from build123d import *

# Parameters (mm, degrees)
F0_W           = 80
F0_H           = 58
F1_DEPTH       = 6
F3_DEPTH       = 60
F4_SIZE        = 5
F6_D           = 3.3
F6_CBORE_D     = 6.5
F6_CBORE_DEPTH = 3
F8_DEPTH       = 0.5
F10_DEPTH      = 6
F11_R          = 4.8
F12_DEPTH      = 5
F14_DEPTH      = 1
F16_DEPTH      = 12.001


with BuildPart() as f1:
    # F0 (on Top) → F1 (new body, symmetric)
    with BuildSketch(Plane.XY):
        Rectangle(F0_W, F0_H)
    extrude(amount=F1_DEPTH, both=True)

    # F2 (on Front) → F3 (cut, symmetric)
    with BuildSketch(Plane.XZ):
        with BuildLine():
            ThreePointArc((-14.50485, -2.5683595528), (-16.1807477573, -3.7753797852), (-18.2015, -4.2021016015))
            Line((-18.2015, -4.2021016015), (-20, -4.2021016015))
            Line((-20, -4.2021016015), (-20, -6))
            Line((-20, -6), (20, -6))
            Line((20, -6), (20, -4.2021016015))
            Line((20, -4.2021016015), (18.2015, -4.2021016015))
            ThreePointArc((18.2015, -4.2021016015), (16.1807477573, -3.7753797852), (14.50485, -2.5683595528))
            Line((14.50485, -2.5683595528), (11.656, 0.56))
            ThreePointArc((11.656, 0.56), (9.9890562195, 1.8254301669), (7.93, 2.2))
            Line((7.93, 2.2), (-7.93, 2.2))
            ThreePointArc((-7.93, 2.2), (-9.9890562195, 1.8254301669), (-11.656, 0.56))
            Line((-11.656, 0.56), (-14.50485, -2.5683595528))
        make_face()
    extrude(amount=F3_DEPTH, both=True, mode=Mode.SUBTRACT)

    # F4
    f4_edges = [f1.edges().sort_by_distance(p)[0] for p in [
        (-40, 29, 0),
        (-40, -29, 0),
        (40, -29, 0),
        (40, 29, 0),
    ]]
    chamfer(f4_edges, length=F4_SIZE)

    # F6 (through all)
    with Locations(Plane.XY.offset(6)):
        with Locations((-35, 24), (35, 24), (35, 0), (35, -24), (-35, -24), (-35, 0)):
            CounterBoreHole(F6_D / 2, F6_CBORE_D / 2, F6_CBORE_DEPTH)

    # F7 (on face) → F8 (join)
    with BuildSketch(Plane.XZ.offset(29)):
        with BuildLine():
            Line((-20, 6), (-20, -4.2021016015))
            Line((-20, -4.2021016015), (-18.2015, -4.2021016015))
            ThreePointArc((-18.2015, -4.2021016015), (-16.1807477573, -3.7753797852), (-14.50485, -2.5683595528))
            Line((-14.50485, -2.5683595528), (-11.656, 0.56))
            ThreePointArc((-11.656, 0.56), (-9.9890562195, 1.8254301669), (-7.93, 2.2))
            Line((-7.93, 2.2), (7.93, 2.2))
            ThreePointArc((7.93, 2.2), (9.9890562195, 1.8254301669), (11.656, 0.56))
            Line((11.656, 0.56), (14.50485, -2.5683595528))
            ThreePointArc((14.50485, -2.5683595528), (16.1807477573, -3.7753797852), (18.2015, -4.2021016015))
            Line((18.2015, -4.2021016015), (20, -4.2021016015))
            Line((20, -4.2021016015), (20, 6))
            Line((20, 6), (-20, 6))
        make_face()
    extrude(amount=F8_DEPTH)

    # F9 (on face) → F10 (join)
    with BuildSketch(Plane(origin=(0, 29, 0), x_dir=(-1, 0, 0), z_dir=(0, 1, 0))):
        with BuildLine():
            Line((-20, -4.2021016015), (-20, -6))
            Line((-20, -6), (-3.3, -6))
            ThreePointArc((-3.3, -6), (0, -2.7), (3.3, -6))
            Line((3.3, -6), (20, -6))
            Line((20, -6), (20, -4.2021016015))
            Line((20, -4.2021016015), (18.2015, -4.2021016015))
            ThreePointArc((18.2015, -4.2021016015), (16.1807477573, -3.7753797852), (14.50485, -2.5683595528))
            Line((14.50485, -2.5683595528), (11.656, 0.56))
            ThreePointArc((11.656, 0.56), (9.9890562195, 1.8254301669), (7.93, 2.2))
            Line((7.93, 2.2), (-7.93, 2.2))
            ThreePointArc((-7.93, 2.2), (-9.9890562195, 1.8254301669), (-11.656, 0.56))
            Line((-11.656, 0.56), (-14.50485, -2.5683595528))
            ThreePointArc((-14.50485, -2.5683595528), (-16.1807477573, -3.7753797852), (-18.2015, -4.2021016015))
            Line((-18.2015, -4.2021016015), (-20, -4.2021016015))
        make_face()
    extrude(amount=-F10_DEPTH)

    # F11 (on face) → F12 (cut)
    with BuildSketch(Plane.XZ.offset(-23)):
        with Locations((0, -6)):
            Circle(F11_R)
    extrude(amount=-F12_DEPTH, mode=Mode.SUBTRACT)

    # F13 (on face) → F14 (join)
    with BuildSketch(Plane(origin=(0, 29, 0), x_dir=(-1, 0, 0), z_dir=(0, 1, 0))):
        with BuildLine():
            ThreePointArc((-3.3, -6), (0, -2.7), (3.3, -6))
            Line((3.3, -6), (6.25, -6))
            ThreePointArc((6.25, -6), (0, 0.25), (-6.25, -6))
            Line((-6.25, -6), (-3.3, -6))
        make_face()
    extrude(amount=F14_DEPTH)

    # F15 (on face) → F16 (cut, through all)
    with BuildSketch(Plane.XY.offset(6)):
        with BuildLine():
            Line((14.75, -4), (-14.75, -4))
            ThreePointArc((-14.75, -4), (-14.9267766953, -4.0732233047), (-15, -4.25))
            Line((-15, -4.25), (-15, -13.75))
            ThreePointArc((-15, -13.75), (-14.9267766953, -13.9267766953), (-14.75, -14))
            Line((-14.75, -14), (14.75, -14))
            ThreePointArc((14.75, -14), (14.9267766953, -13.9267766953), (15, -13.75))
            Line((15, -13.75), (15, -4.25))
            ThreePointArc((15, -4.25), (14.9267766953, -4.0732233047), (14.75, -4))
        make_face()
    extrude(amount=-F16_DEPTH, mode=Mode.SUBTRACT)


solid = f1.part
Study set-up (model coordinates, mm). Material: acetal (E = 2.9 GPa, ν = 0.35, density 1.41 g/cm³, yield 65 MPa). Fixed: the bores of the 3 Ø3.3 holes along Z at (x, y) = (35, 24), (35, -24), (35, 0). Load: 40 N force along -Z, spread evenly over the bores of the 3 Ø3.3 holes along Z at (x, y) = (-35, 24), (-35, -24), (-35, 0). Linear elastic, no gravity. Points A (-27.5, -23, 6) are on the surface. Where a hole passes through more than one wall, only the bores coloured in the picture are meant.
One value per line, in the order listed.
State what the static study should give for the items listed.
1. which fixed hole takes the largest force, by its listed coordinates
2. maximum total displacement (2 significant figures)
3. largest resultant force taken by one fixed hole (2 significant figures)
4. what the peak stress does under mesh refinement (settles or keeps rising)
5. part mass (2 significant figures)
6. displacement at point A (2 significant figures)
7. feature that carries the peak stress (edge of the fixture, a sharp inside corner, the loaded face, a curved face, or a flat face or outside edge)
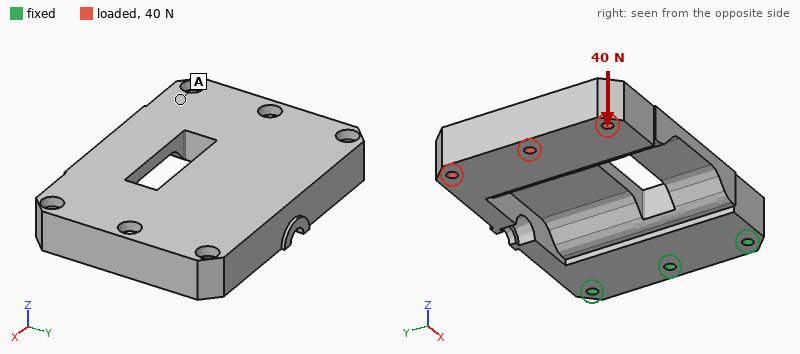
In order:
(35, 0)
1.2 mm
49 N
keeps rising
57 g
0.83 mm
a sharp inside corner
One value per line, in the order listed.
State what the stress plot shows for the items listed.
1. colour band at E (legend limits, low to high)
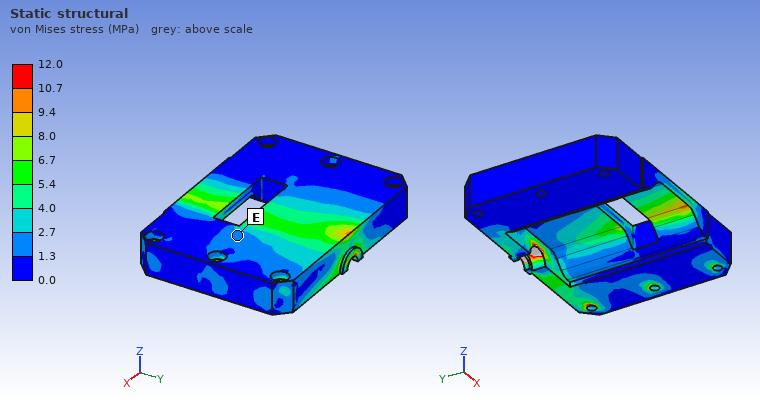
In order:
1.3 to 2.7 MPa
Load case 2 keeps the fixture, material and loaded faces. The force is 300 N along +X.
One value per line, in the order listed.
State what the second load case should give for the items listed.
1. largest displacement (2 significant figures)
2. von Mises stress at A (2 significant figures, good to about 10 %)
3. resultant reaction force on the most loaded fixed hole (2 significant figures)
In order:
0.94 mm
1.0 MPa
120 N
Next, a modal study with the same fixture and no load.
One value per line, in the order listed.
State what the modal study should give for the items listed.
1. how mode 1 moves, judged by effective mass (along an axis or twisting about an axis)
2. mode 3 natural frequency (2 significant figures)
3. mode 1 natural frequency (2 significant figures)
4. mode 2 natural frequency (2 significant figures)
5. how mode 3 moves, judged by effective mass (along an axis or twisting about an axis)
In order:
along Z
1300 Hz
250 Hz
720 Hz
along Y
